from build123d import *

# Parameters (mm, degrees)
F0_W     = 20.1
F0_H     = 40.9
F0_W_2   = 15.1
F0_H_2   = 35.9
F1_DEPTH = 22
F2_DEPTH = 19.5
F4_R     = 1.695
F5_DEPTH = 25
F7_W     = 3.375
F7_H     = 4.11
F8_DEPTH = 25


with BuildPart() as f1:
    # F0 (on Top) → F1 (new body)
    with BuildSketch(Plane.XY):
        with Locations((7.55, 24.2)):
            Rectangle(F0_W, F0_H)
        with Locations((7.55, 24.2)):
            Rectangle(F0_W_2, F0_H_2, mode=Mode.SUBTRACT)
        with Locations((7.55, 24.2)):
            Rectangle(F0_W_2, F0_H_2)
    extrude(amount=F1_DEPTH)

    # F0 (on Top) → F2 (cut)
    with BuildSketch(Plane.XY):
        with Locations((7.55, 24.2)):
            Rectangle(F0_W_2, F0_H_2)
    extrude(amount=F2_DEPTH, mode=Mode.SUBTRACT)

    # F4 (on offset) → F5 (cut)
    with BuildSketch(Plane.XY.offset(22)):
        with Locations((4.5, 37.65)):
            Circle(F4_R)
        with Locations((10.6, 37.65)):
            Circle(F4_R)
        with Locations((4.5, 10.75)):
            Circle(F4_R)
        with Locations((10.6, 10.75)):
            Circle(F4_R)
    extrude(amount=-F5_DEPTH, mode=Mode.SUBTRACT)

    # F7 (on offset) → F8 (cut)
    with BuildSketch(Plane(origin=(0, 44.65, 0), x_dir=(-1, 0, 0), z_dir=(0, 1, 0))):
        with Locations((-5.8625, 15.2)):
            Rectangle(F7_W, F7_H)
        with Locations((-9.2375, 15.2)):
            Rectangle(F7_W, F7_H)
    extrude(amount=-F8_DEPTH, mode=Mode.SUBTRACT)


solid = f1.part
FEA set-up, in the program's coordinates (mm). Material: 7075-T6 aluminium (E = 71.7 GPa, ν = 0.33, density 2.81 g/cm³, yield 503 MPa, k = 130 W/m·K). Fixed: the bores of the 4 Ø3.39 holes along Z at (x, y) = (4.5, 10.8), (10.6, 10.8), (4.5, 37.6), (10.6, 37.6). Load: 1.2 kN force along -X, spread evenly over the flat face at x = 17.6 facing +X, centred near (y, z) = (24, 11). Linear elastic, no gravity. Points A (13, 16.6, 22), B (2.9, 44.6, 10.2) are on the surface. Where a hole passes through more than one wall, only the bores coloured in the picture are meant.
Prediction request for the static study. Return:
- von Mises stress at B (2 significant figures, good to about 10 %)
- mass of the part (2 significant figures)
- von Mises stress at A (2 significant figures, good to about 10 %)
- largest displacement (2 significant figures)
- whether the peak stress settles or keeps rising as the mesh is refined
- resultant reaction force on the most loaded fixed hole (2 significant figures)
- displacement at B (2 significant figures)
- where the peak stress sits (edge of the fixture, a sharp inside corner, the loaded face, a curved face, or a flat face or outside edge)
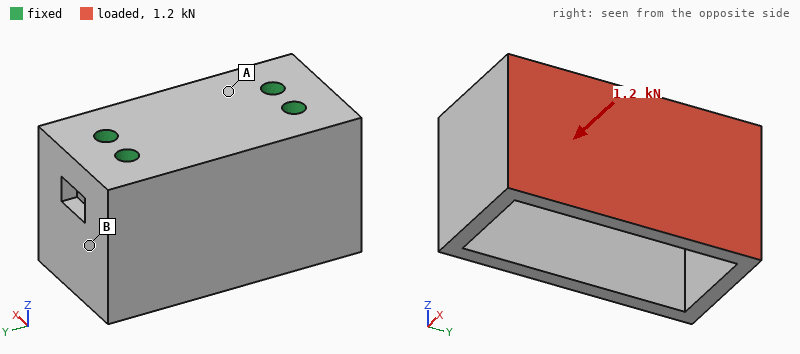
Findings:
17 MPa
21 g
47 MPa
0.14 mm
keeps rising
640 N
0.027 mm
edge of the fixture
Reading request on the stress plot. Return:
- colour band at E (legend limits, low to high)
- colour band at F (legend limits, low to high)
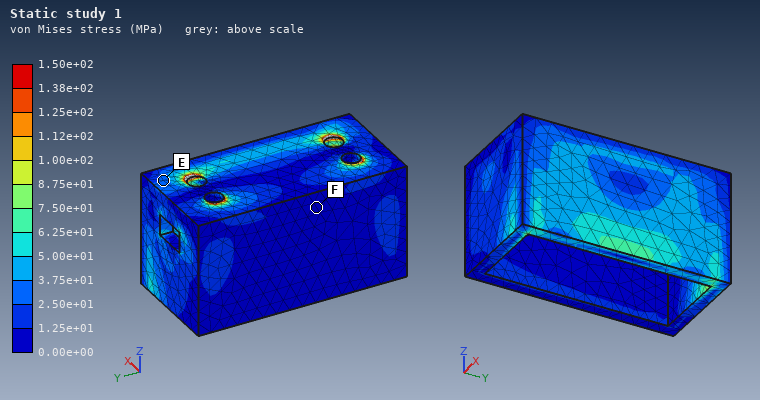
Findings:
2.50e+01 to 3.75e+01 MPa
0.00e+00 to 1.25e+01 MPa
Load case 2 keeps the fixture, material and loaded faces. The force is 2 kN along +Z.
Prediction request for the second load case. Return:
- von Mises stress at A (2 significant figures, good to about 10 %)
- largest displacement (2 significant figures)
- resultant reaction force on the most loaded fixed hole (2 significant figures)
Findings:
48 MPa
98 µm
1.4 kN
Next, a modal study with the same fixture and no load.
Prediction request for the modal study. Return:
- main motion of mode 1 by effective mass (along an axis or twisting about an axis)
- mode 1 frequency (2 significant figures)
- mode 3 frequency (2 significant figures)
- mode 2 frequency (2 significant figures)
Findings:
along X
6300 Hz
8800 Hz
8200 Hz
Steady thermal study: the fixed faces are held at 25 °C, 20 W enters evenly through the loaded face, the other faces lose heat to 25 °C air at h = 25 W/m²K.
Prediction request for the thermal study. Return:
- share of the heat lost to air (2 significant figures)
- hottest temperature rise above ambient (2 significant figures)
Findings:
4.2 %
18 K
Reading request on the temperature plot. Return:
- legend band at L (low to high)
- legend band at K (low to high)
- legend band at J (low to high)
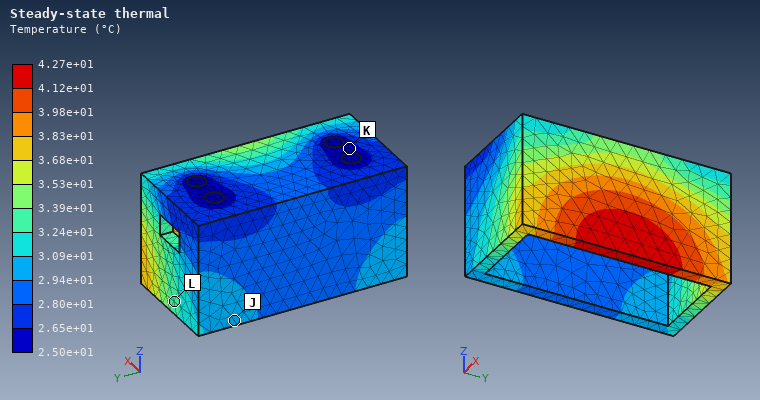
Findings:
3.24e+01 to 3.39e+01 °C
2.50e+01 to 2.65e+01 °C
2.94e+01 to 3.09e+01 °C
